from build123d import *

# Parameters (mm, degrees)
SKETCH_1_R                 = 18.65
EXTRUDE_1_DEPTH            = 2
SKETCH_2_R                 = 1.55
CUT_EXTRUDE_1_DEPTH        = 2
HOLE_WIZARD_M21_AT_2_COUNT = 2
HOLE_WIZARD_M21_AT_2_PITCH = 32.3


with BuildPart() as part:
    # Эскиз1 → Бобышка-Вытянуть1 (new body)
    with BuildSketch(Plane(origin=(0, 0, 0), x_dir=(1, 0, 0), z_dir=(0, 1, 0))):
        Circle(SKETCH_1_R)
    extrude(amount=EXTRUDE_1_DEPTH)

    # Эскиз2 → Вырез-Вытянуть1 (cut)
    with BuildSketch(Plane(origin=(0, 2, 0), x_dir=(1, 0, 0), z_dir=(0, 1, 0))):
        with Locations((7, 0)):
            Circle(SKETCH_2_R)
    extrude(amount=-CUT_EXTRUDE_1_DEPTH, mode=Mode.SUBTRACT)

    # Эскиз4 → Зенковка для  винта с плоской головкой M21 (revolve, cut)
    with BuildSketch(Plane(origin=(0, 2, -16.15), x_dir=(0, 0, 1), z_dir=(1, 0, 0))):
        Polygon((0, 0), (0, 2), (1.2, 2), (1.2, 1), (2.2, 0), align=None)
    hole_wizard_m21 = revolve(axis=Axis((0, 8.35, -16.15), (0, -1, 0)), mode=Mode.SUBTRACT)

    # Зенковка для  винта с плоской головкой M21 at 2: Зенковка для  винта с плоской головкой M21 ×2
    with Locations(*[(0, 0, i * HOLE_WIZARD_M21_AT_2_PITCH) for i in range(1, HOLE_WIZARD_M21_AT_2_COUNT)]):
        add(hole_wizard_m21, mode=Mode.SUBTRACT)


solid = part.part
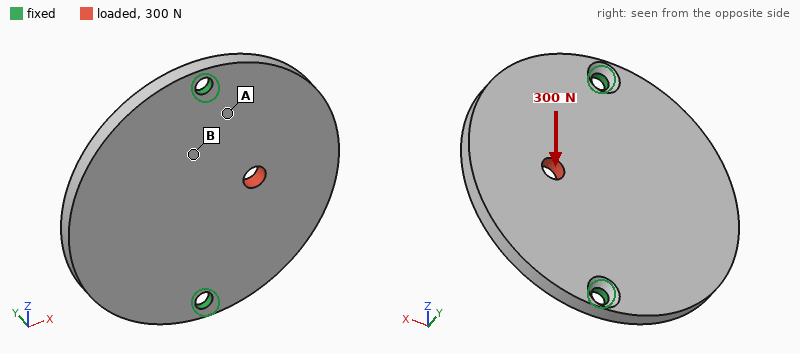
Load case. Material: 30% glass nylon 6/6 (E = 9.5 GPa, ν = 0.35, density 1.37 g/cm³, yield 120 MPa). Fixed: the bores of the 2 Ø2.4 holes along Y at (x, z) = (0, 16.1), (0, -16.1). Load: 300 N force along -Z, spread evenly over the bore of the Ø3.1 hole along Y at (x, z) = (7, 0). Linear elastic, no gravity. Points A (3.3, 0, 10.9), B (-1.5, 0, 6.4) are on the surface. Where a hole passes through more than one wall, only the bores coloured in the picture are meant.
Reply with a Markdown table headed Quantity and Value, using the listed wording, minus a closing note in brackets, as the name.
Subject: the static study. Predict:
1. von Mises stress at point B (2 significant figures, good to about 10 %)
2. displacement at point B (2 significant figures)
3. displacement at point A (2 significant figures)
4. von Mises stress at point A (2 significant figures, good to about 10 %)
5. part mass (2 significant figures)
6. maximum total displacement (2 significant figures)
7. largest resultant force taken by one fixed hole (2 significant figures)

| Quantity | Value |
|---|---|
| von Mises stress at point B | 5.0 MPa |
| displacement at point B | 9.1 µm |
| displacement at point A | 11 µm |
| von Mises stress at point A | 11 MPa |
| part mass | 2.9 g |
| maximum total displacement | 24 µm |
| largest resultant force taken by one fixed hole | 160 N |
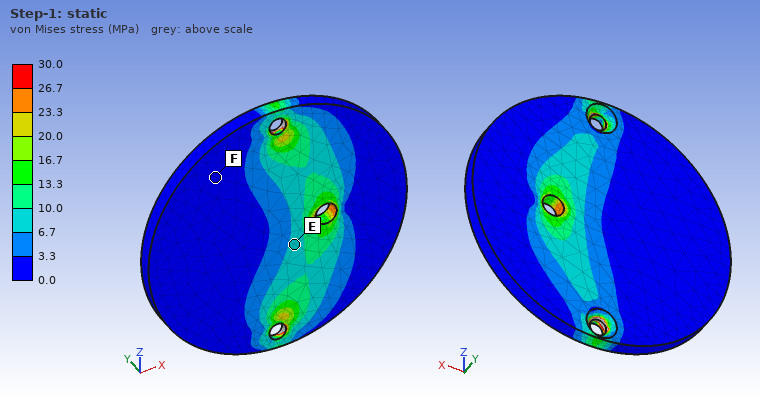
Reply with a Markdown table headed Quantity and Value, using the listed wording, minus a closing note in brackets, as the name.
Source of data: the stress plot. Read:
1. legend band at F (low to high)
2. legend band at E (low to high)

| Quantity | Value |
|---|---|
| legend band at F | 0.0 to 3.3 MPa |
| legend band at E | 6.7 to 10.0 MPa |
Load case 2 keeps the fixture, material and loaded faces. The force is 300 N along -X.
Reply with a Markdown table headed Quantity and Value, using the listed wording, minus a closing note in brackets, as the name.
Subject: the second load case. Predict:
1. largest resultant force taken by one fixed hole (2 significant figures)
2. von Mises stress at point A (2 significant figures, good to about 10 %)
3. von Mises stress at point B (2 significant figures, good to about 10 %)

| Quantity | Value |
|---|---|
| largest resultant force taken by one fixed hole | 150 N |
| von Mises stress at point A | 5.9 MPa |
| von Mises stress at point B | 4.6 MPa |
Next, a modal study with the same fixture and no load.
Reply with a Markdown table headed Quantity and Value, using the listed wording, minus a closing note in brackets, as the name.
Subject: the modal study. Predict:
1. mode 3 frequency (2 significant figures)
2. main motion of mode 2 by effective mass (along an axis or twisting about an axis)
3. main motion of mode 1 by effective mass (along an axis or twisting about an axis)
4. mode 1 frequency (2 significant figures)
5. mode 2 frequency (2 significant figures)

| Quantity | Value |
|---|---|
| mode 3 frequency | 5200 Hz |
| main motion of mode 2 by effective mass | along Y |
| main motion of mode 1 by effective mass | twisting about Z |
| mode 1 frequency | 1500 Hz |
| mode 2 frequency | 2400 Hz |
